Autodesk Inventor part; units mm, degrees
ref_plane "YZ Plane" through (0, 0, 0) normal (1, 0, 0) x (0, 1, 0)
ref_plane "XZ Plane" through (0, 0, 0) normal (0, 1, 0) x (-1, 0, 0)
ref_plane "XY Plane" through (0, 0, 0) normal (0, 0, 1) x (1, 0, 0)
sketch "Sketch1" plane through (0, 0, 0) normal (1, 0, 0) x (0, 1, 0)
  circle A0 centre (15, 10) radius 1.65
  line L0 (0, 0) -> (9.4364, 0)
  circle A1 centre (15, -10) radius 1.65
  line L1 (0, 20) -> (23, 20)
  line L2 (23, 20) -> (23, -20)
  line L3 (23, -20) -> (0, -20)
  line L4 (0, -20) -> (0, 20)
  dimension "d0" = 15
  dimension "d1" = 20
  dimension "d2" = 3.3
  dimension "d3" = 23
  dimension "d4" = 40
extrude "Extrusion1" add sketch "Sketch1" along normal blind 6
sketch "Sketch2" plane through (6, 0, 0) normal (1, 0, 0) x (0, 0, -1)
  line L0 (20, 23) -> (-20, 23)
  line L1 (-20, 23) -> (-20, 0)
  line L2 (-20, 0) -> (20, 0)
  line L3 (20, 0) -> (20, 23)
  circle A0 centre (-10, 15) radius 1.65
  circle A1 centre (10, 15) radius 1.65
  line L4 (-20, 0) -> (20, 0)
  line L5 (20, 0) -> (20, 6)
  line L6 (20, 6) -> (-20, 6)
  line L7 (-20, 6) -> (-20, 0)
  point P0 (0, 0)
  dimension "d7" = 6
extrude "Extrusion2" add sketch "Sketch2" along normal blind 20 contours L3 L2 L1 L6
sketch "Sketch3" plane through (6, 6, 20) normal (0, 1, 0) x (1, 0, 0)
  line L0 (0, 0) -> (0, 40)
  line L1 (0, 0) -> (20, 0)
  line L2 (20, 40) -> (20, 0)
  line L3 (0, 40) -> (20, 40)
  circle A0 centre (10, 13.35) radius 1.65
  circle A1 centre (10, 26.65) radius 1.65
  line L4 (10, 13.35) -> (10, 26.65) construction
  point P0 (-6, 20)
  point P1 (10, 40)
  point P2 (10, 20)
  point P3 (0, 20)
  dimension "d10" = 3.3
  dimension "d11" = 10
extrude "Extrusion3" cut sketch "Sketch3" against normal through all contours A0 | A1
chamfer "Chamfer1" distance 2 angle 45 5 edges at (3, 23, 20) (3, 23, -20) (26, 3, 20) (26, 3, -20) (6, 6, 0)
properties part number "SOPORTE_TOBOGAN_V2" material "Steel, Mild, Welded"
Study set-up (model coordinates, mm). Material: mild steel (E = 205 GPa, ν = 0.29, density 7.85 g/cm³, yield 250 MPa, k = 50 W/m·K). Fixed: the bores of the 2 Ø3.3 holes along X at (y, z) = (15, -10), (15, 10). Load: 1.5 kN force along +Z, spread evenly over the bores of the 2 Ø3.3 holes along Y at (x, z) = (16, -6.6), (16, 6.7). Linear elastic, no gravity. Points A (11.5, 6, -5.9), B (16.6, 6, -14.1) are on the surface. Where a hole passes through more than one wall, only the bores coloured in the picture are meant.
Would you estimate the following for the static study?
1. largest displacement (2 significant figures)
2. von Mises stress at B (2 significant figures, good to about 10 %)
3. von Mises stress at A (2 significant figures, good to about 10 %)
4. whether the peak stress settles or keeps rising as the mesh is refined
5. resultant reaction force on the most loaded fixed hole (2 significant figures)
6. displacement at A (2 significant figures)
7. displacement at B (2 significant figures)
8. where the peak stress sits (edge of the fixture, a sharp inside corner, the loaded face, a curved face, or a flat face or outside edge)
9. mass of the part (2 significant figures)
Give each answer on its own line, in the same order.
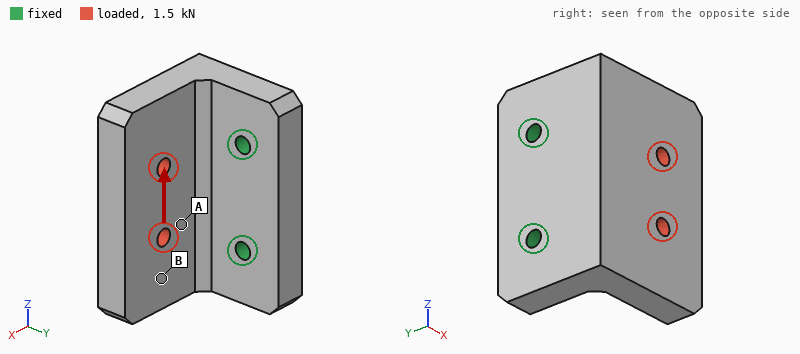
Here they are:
13 µm
12 MPa
29 MPa
keeps rising
1.3 kN
5.3 µm
8.7 µm
edge of the fixture
80 g
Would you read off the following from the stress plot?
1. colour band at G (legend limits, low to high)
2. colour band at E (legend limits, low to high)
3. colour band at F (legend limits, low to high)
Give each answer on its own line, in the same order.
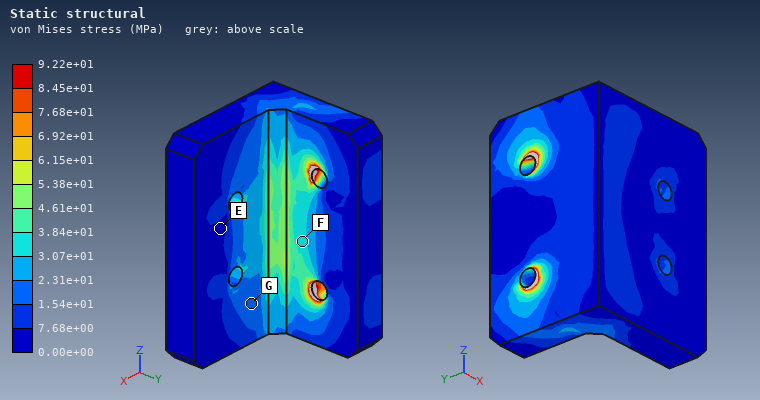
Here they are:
1.54e+01 to 2.31e+01 MPa
0.00e+00 to 7.68e+00 MPa
3.07e+01 to 3.84e+01 MPa
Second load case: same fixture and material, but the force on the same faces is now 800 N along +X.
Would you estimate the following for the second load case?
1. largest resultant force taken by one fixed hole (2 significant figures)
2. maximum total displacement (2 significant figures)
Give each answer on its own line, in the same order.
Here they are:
400 N
13 µm
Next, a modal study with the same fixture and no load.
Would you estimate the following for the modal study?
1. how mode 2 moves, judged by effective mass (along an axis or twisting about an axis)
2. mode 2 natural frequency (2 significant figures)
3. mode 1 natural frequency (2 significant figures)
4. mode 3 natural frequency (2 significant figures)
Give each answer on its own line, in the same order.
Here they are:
along Z
8800 Hz
5200 Hz
14 kHz
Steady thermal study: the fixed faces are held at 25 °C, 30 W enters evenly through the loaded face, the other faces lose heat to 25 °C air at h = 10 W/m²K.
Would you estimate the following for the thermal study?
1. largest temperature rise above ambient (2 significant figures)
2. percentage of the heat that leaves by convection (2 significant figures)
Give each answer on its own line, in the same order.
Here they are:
67 K
4.5 %
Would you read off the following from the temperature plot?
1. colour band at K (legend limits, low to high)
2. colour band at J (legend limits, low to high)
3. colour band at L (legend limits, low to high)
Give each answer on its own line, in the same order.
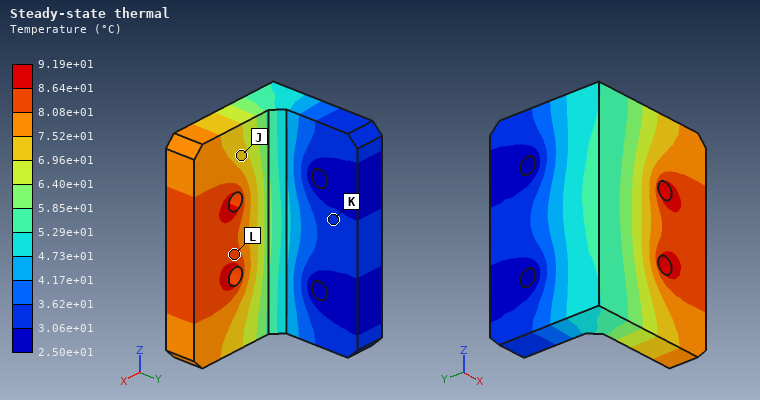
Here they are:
3.06e+01 to 3.62e+01 °C
6.96e+01 to 7.52e+01 °C
8.08e+01 to 8.64e+01 °C
